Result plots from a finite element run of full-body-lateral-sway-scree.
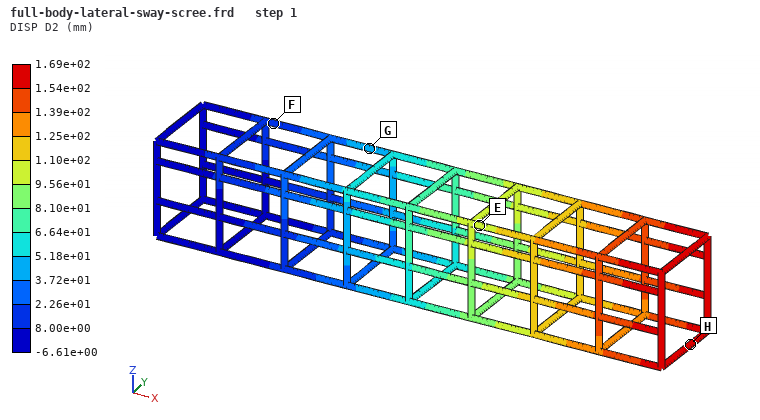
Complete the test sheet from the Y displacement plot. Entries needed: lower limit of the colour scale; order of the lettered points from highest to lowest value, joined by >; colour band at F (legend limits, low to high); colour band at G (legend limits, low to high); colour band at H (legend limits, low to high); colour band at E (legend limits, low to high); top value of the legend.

-6.61e+00 mm
H > E > G > F
8.00e+00 to 2.26e+01 mm
3.72e+01 to 5.18e+01 mm
1.54e+02 to 1.69e+02 mm
9.56e+01 to 1.10e+02 mm
1.69e+02 mm
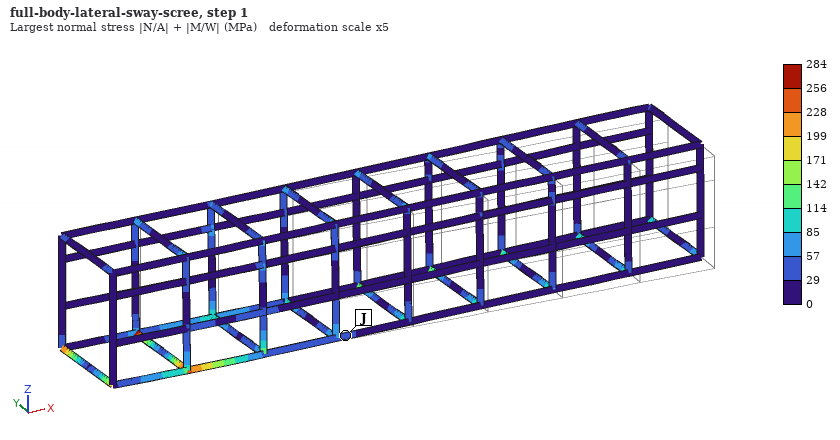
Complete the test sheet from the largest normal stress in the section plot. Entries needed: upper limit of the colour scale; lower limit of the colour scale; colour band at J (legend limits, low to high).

284 MPa
0 MPa
29 to 57 MPa
